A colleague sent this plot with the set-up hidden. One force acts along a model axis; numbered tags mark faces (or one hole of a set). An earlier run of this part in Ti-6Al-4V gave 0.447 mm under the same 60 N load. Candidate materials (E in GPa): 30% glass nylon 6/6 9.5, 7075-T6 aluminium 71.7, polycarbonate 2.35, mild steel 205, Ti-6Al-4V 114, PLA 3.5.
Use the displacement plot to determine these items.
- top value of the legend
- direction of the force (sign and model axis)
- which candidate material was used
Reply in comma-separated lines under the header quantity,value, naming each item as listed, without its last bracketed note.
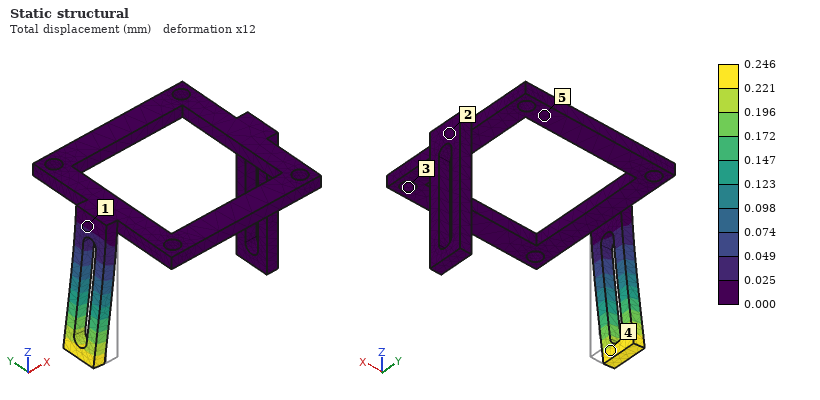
quantity,value
top value of the legend,0.246 mm
direction of the force,-X
which candidate material was used,mild steel
